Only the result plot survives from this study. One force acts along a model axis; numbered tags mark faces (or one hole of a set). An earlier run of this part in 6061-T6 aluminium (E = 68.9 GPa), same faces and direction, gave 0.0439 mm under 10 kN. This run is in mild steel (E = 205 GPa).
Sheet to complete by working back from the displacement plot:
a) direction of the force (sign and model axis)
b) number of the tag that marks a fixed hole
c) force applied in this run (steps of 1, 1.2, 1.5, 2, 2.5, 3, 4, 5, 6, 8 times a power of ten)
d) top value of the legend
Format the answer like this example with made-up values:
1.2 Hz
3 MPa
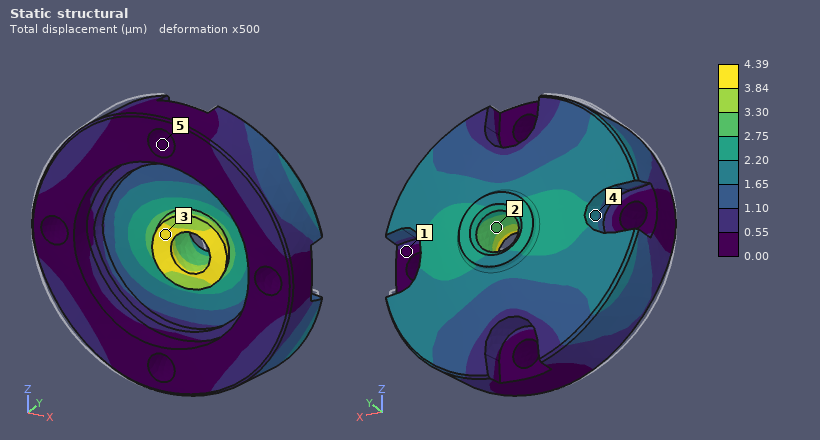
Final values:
+X
5
3 kN
4.39 µm
